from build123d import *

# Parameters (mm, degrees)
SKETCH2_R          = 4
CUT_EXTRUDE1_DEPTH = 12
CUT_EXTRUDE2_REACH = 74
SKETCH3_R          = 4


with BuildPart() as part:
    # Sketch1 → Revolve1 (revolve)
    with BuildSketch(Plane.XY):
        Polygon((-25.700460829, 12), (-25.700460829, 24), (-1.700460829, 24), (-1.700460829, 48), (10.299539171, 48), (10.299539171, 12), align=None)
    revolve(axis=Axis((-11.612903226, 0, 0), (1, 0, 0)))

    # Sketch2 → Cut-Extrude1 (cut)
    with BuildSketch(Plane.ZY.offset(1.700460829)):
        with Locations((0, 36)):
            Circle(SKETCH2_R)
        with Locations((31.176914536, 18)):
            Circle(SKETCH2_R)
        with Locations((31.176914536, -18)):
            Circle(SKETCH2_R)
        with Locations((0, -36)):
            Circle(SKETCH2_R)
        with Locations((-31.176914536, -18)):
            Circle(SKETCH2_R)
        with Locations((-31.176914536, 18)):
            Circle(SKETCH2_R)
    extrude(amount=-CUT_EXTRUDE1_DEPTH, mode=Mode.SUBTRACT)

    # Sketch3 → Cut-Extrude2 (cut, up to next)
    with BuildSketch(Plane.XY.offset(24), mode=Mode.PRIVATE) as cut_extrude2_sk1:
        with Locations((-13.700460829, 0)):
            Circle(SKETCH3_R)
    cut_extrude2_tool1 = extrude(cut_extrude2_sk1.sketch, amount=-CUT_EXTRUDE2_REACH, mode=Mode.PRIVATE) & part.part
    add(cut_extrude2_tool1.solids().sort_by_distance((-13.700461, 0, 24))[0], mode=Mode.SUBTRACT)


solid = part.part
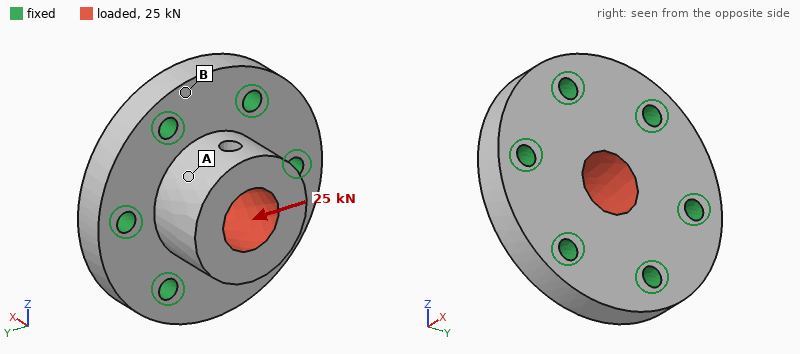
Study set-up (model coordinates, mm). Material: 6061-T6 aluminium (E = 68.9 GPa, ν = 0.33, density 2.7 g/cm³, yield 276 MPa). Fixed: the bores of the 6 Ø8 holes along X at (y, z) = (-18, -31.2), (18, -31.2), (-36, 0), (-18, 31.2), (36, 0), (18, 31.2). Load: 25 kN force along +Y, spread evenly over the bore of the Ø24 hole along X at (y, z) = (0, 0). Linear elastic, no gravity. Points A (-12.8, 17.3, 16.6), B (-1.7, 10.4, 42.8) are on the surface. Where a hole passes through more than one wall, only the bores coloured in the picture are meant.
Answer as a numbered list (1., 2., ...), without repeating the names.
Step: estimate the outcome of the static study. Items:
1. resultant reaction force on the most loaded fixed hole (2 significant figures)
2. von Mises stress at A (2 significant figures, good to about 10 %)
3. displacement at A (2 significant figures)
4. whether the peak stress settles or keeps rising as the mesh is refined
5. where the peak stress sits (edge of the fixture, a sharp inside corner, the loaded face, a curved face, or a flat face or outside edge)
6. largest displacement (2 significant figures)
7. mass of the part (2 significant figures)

1. 6.9 kN
2. 13 MPa
3. 17 µm
4. keeps rising
5. edge of the fixture
6. 29 µm
7. 300 g
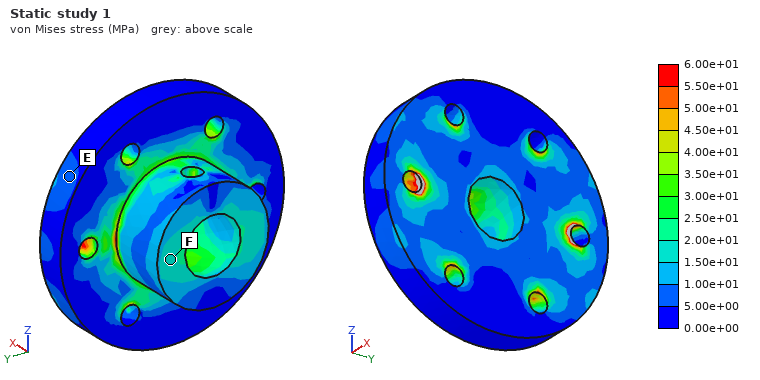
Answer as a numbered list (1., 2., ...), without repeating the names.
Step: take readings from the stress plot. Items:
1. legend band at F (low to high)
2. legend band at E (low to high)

1. 1.50e+01 to 2.00e+01 MPa
2. 5.00e+00 to 1.00e+01 MPa
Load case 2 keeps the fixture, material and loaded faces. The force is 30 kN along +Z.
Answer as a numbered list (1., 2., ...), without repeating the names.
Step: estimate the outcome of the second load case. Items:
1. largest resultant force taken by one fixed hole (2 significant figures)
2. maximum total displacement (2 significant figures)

1. 7.3 kN
2. 34 µm
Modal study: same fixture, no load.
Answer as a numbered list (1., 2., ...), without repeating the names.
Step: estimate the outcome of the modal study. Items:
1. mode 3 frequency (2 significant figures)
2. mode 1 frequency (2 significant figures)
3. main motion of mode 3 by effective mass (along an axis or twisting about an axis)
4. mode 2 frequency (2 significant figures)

1. 16 kHz
2. 15 kHz
3. along X
4. 15 kHz
